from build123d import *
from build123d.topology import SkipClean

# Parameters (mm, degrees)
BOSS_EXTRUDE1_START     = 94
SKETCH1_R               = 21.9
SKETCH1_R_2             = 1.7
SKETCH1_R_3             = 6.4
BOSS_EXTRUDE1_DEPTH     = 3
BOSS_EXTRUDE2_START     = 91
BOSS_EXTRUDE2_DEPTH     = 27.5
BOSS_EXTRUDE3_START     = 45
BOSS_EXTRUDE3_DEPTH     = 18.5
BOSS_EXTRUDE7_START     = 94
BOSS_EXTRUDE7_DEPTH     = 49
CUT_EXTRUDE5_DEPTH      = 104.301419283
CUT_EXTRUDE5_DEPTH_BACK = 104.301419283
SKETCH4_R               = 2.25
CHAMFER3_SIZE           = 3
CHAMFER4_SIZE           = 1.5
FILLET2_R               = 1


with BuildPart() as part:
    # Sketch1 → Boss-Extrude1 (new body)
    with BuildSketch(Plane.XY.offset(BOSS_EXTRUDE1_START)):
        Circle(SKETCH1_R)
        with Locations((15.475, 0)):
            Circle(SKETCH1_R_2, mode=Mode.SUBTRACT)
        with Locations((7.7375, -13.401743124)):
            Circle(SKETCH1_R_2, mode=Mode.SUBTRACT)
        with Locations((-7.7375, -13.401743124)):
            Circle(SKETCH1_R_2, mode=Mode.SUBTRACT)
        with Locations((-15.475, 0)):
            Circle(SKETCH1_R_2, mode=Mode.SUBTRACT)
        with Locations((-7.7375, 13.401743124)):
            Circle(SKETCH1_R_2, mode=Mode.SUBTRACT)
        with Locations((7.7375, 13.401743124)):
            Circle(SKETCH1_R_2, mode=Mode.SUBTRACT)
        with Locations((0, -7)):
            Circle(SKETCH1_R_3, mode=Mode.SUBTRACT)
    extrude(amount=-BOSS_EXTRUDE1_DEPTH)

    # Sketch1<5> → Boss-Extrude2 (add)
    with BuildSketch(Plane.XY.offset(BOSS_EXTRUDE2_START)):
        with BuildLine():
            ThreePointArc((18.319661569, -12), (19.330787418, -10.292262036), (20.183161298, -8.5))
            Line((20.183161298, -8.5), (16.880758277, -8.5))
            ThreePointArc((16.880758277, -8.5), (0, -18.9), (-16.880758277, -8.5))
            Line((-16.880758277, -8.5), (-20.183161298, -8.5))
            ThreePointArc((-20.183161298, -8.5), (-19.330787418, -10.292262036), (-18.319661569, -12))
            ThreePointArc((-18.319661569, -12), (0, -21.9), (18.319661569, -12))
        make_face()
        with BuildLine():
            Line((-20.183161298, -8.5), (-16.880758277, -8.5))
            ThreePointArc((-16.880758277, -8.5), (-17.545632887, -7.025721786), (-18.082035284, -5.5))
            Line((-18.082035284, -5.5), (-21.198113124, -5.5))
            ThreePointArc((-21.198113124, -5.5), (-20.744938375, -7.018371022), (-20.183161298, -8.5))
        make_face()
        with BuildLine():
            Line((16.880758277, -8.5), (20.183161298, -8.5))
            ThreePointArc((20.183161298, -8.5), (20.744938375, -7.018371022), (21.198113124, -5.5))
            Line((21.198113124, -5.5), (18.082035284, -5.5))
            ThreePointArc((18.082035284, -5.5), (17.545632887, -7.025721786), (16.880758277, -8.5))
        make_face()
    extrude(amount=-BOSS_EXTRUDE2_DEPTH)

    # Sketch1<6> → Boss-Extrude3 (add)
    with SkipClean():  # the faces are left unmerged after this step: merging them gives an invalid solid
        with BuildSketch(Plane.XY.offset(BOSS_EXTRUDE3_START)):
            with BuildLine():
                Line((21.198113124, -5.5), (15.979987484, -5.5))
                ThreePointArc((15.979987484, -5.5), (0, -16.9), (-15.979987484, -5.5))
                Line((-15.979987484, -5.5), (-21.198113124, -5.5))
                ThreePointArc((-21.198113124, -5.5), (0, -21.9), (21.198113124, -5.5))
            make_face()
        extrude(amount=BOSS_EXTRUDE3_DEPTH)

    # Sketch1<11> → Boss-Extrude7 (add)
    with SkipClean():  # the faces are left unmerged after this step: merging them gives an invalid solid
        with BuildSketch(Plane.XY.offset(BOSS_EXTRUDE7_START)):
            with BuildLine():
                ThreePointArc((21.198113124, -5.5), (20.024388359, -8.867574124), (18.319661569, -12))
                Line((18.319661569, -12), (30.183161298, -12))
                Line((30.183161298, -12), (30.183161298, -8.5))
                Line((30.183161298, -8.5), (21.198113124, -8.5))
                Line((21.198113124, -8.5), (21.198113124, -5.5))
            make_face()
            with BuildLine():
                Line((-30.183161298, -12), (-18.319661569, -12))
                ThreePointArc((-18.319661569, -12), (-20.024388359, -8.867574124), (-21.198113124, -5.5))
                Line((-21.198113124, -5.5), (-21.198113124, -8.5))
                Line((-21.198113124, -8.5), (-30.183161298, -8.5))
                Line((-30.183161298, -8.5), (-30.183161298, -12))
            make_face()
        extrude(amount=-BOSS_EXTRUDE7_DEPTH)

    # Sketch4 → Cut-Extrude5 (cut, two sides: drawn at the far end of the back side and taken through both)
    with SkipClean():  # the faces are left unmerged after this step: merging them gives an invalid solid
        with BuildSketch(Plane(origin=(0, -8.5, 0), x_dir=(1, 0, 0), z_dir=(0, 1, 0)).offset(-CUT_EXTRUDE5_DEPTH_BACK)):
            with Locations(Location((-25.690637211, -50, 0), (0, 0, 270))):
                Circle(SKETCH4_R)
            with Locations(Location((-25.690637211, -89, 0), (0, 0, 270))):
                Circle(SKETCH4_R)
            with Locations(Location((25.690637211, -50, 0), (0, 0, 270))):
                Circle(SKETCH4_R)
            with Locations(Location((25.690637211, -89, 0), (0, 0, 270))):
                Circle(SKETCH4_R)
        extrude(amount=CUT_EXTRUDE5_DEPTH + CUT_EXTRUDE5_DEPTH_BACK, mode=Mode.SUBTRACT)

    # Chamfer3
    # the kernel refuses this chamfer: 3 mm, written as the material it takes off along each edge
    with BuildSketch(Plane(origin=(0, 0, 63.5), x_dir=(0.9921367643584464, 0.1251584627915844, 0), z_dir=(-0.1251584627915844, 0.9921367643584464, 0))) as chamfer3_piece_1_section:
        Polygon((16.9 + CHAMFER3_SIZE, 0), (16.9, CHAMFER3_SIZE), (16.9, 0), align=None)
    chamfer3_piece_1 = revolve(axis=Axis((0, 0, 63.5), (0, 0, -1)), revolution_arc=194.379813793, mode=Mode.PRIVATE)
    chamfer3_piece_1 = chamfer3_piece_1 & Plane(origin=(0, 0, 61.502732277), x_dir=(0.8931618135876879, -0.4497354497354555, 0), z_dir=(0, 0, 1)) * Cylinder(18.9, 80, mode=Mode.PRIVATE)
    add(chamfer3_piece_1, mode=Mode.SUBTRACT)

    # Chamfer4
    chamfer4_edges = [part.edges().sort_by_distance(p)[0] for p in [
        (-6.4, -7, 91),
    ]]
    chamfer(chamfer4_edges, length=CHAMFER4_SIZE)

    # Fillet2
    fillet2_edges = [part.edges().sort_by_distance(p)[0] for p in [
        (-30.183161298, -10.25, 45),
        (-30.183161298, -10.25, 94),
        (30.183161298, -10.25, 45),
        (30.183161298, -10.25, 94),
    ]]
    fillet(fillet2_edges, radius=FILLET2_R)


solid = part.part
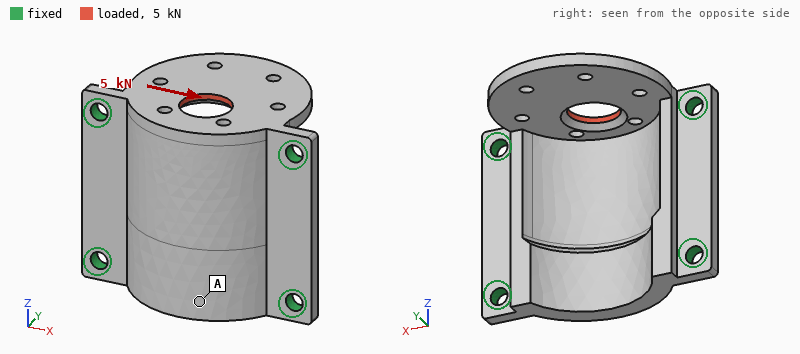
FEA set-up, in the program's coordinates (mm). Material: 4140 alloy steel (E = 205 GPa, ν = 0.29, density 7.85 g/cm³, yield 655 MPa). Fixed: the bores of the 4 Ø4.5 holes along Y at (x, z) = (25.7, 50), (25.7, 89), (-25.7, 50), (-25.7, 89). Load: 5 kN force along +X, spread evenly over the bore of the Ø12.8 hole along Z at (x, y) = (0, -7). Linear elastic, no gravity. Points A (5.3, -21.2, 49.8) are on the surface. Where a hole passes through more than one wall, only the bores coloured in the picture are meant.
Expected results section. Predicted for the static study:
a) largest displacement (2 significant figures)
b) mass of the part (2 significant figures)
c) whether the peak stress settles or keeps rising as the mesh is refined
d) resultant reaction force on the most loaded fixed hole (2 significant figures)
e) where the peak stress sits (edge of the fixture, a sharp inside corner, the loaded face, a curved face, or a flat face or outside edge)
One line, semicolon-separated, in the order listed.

11 µm; 130 g; keeps rising; 2.4 kN; edge of the fixture
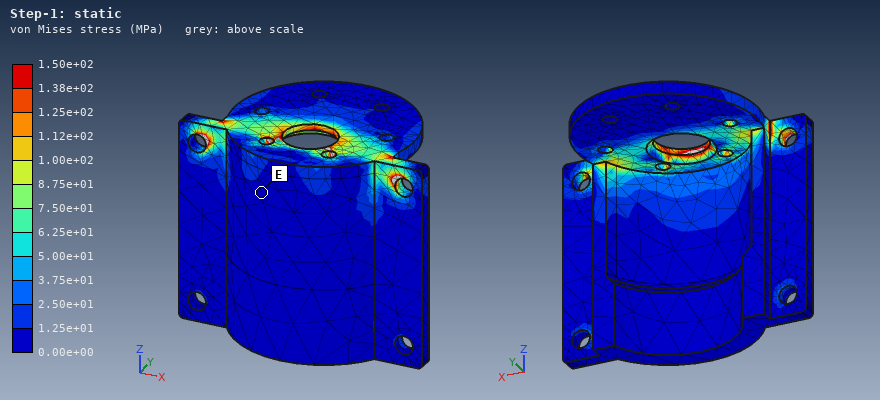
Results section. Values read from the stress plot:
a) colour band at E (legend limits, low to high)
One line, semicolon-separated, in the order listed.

0.00e+00 to 1.25e+01 MPa
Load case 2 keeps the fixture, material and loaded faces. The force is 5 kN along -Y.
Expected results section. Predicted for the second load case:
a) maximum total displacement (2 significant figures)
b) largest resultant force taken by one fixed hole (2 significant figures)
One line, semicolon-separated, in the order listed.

99 µm; 2.7 kN
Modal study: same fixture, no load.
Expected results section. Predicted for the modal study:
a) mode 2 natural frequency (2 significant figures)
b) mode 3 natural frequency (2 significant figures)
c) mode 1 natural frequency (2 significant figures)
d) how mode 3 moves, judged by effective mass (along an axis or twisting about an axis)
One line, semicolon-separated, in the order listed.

7000 Hz; 11 kHz; 2400 Hz; along Y
